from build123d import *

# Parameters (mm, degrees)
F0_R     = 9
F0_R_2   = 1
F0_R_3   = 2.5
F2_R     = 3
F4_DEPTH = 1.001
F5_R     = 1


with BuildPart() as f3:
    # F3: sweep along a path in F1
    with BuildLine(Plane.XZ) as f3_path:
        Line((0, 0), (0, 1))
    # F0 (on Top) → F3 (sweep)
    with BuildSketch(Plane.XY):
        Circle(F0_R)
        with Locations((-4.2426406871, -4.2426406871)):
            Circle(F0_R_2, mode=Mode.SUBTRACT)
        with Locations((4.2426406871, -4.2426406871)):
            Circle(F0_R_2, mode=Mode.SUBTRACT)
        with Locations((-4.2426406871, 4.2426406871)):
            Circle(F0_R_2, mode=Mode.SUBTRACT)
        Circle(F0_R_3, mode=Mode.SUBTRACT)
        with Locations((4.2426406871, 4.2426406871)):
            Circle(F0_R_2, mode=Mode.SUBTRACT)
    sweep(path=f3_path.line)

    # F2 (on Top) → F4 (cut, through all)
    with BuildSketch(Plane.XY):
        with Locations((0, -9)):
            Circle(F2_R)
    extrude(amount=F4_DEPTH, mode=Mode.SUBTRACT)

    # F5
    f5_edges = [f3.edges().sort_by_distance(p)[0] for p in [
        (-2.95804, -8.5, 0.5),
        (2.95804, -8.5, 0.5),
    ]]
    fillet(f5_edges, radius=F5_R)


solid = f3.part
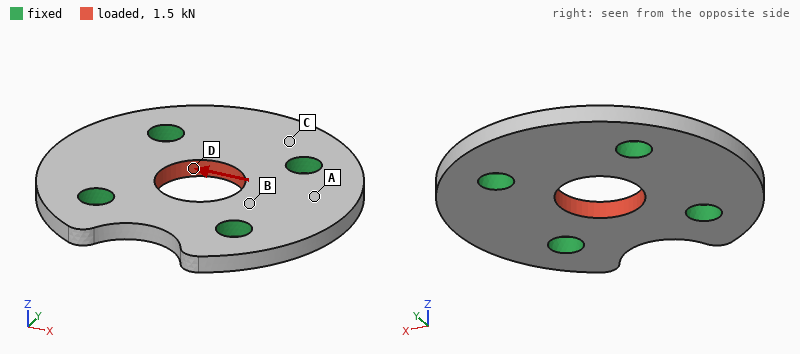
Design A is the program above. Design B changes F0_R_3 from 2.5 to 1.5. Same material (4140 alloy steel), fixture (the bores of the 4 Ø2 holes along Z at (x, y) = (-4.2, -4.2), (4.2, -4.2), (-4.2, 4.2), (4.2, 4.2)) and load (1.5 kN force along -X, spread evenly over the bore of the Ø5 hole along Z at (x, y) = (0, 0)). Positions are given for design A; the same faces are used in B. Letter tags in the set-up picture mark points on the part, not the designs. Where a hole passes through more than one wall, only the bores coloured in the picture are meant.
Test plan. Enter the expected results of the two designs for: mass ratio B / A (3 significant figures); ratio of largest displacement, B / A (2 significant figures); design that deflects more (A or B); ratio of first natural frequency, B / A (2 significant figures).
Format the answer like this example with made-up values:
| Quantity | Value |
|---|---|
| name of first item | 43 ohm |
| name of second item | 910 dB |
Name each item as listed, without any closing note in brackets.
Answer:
| Quantity | Value |
|---|---|
| mass ratio B / A | 1.06 |
| ratio of largest displacement, B / A | 1.3 |
| design that deflects more | B |
| ratio of first natural frequency, B / A | 1.0 |
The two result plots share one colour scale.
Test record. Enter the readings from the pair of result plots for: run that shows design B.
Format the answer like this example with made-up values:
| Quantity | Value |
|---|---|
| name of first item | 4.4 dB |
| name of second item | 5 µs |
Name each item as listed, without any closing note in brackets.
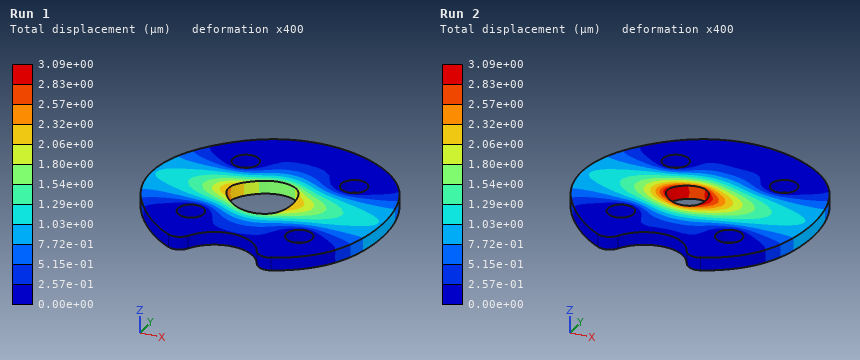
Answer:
| Quantity | Value |
|---|---|
| run that shows design B | Run 2 |
